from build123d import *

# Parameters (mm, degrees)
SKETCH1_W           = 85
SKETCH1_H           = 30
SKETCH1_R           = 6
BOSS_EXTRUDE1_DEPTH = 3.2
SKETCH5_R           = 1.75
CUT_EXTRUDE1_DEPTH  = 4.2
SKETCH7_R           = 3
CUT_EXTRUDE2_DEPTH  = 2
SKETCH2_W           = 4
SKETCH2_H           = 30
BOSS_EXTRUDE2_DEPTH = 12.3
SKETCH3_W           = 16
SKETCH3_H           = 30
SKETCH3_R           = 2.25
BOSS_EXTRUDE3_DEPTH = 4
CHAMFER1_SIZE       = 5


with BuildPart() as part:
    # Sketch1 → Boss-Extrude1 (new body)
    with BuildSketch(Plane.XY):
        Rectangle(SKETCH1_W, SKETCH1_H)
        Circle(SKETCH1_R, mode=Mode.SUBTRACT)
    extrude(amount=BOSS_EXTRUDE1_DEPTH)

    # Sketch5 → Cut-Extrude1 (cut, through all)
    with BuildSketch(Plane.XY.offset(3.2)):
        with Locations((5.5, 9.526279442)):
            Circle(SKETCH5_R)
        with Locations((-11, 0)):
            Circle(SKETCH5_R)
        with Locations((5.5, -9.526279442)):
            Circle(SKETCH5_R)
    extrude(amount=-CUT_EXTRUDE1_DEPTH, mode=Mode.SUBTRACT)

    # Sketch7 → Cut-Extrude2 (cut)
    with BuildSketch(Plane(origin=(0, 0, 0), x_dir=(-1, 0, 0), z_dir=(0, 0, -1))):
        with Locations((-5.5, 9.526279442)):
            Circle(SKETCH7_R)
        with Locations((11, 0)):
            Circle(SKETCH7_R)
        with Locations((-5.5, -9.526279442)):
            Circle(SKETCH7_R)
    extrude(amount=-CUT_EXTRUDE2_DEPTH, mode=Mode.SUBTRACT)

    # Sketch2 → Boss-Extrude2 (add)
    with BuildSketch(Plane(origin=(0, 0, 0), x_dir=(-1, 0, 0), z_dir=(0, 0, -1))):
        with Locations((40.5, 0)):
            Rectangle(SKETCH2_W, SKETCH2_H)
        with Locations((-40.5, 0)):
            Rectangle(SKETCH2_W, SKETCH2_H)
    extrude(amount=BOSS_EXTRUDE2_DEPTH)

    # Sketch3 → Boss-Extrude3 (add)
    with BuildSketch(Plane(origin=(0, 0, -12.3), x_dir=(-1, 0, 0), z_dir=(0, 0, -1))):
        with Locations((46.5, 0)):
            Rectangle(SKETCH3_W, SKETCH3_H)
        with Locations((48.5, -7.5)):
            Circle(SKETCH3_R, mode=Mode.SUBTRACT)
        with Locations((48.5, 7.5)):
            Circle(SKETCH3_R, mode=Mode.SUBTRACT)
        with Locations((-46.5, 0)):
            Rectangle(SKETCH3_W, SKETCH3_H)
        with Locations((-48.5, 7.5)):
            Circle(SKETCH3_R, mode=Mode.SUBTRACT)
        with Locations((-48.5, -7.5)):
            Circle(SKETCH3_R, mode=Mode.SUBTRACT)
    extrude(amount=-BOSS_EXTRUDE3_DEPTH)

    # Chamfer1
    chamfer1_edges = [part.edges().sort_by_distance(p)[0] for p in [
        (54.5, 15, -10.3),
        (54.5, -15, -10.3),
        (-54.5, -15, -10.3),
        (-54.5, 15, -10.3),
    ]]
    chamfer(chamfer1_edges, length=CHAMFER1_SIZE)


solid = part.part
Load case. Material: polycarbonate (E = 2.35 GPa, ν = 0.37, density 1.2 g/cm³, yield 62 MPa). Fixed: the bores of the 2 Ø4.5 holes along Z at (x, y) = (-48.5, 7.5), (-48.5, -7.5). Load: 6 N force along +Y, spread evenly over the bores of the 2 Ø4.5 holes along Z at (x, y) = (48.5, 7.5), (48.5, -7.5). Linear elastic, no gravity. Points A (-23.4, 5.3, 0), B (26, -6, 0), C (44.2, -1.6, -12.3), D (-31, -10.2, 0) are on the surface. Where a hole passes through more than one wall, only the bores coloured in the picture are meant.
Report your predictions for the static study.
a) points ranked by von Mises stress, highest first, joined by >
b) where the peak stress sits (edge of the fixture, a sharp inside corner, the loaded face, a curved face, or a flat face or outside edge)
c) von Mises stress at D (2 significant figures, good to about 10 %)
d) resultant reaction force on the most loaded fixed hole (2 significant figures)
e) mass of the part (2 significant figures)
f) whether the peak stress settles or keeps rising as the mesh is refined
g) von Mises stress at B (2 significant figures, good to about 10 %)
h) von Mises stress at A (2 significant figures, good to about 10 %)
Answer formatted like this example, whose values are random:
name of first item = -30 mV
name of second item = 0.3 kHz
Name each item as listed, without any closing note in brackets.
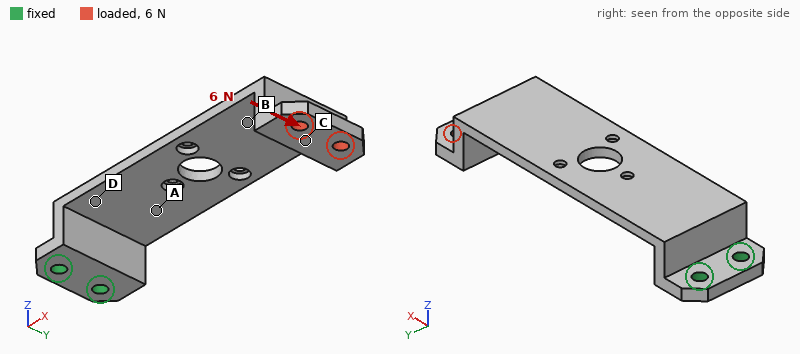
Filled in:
points ranked by von Mises stress, highest first, joined by > = D > A > B > C
where the peak stress sits = edge of the fixture
von Mises stress at D = 2.2 MPa
resultant reaction force on the most loaded fixed hole = 32 N
mass of the part = 16 g
whether the peak stress settles or keeps rising as the mesh is refined = keeps rising
von Mises stress at B = 1.3 MPa
von Mises stress at A = 1.7 MPa
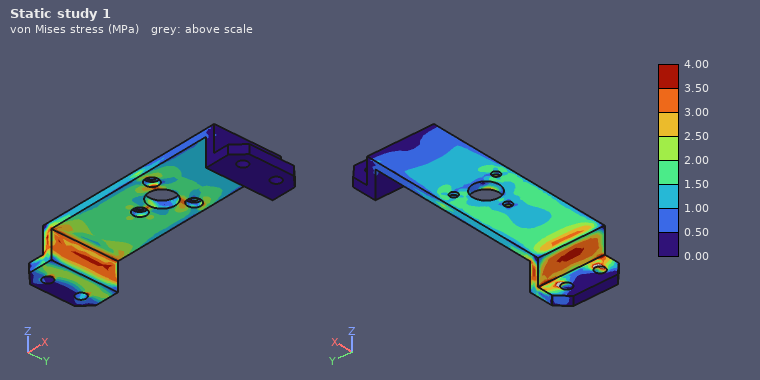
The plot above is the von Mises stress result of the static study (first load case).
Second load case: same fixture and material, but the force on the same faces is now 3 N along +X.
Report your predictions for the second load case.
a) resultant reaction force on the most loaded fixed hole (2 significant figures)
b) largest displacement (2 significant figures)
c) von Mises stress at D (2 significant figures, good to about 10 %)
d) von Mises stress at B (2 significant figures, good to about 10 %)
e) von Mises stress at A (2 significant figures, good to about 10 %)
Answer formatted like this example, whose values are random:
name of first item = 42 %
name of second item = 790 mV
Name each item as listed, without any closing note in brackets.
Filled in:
resultant reaction force on the most loaded fixed hole = 1.5 N
largest displacement = 1.0 mm
von Mises stress at D = 0.70 MPa
von Mises stress at B = 0.69 MPa
von Mises stress at A = 0.69 MPa
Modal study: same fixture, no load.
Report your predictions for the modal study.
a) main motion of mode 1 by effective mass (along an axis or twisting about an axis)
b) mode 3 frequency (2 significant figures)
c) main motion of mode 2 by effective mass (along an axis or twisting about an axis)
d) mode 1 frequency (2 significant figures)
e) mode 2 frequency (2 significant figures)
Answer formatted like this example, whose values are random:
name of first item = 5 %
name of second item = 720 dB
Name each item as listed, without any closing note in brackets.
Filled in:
main motion of mode 1 by effective mass = along Z
mode 3 frequency = 340 Hz
main motion of mode 2 by effective mass = along Y
mode 1 frequency = 57 Hz
mode 2 frequency = 190 Hz
